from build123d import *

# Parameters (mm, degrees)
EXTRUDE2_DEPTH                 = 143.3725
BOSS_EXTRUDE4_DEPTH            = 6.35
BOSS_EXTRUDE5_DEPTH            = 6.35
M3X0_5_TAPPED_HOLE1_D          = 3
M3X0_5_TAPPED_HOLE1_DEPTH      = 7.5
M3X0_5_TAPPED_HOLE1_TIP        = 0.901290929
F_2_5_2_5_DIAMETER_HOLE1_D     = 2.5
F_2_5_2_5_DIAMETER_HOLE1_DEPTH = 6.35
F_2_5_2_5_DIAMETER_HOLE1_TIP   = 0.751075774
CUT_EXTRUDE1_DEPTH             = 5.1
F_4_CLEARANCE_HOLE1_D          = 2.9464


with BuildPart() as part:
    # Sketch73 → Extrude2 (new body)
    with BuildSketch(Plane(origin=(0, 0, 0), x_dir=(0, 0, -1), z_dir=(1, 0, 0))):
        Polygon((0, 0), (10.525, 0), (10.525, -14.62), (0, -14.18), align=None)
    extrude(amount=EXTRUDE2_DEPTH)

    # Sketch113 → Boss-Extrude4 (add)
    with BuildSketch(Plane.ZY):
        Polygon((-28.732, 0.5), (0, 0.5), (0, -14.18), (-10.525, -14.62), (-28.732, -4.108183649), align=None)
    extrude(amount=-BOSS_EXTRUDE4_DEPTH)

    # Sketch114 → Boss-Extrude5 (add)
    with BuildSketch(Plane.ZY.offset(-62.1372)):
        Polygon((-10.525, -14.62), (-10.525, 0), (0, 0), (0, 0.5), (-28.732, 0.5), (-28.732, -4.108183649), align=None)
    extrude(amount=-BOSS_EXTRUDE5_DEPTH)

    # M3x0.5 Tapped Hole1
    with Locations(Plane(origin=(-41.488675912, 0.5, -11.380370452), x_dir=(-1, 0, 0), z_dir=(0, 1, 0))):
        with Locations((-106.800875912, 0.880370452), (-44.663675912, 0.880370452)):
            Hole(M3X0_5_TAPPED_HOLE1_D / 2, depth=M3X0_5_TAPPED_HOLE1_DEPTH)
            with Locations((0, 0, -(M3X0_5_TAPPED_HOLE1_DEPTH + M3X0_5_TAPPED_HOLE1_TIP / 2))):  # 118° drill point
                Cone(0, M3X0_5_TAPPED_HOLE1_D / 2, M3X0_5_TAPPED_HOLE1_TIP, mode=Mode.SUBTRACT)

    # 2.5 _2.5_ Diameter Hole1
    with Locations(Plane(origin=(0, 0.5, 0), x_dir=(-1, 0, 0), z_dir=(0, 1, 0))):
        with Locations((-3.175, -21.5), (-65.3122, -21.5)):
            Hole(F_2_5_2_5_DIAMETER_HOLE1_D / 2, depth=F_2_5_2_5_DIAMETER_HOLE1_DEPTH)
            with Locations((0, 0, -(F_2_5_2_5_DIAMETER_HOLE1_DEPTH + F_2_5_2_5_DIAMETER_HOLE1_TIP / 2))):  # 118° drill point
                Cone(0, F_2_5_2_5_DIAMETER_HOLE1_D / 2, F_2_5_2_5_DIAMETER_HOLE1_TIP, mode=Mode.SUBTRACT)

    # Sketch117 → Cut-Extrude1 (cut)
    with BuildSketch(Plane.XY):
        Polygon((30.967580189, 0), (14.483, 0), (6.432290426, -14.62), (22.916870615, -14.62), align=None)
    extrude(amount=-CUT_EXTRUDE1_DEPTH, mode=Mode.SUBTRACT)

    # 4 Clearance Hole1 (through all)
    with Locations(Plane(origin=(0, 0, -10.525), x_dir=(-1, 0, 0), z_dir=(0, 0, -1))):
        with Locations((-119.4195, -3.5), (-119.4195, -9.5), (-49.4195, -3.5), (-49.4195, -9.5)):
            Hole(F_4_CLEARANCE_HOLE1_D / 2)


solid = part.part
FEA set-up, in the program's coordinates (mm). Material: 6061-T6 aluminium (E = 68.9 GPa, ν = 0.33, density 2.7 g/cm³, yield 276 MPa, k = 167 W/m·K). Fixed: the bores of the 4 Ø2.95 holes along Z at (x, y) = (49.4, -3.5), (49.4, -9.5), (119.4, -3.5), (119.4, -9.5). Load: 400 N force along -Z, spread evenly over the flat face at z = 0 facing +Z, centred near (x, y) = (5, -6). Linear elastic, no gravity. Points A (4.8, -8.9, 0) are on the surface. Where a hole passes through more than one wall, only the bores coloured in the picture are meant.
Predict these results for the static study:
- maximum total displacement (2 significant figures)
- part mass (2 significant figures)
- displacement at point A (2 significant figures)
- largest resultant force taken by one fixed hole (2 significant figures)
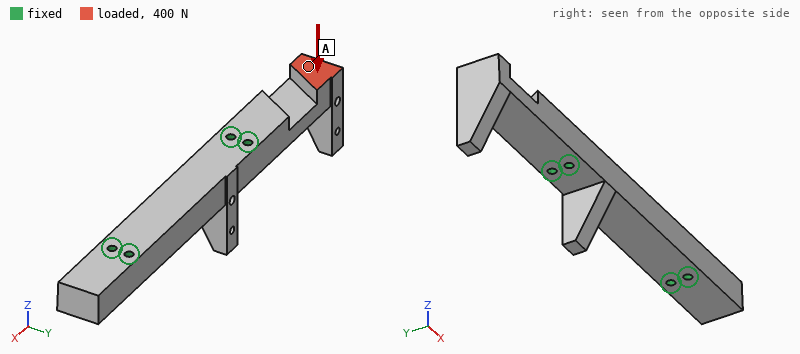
0.37 mm
61 g
0.24 mm
210 N
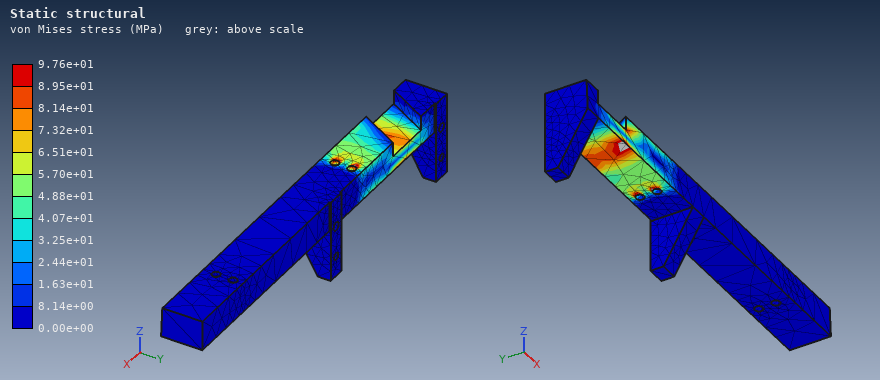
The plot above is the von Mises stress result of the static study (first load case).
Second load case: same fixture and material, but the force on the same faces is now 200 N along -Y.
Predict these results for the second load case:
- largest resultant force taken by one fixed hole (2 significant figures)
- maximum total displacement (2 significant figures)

1.0 kN
69 µm
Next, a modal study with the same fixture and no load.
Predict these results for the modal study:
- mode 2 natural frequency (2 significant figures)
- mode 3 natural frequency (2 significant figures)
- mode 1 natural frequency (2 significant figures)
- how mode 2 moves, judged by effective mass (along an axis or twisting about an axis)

3400 Hz
6100 Hz
2100 Hz
along Y
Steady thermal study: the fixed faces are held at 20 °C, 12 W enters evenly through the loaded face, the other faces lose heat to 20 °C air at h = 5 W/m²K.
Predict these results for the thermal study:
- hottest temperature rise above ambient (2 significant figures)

31 K
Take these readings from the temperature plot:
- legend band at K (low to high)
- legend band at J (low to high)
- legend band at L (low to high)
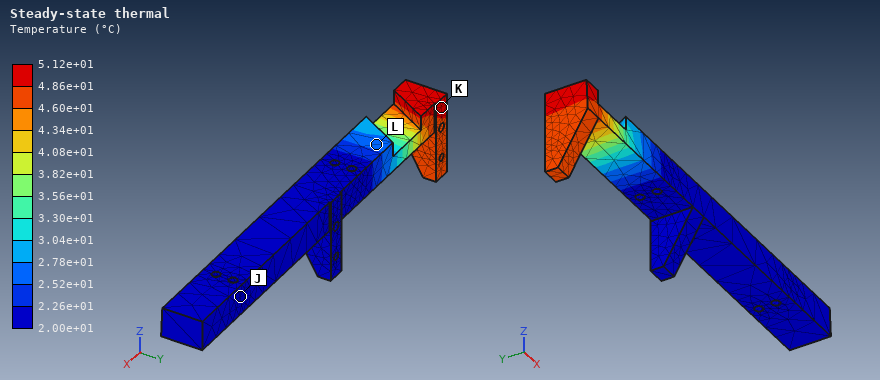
4.86e+01 to 5.12e+01 °C
2.00e+01 to 2.26e+01 °C
2.52e+01 to 2.78e+01 °C
